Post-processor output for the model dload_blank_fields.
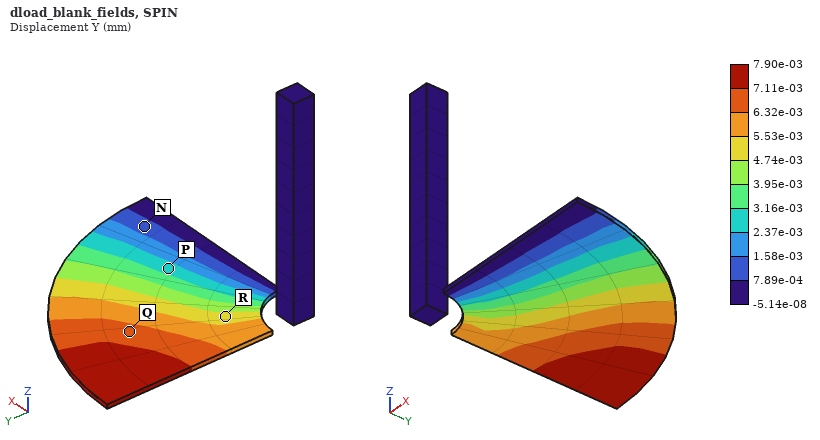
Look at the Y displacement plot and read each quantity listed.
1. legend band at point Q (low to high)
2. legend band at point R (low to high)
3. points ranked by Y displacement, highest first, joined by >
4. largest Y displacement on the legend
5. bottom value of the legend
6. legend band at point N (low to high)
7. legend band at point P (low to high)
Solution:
6.32e-03 to 7.11e-03 mm
4.74e-03 to 5.53e-03 mm
Q > R > P > N
7.90e-03 mm
-5.14e-08 mm
7.89e-04 to 1.58e-03 mm
2.37e-03 to 3.16e-03 mm
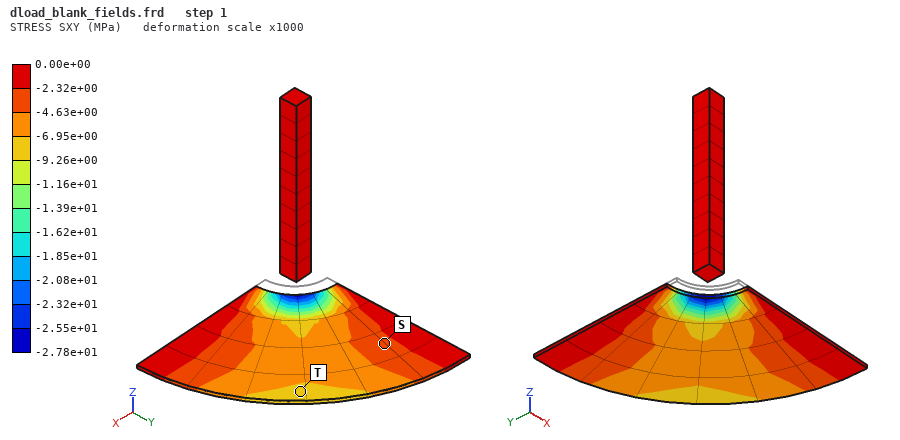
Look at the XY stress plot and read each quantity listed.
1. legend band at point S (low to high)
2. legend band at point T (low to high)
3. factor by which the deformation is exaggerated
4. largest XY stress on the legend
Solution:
-4.63e+00 to -2.32e+00 MPa
-9.26e+00 to -6.95e+00 MPa
1000
0.00e+00 MPa
